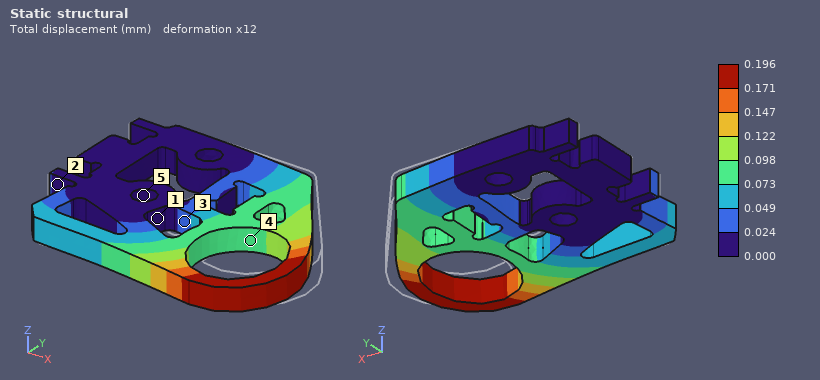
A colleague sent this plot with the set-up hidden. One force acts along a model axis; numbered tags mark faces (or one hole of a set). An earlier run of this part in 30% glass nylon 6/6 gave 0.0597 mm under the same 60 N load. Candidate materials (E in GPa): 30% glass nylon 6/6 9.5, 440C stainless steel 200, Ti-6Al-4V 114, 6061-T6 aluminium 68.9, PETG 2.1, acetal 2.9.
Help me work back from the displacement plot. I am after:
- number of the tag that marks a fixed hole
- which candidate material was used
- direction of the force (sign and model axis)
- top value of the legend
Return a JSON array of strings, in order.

["5", "acetal", "-Y", "0.196 mm"]
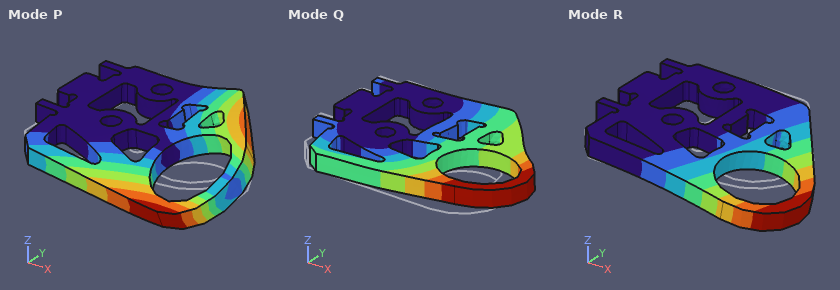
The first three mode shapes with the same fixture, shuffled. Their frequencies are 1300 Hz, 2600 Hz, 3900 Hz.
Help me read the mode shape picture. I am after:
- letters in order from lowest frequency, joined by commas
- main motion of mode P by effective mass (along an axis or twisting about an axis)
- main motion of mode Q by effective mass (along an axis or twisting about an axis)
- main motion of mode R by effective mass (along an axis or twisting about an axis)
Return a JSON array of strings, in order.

["R, P, Q", "twisting about X", "along Y", "along Z"]
